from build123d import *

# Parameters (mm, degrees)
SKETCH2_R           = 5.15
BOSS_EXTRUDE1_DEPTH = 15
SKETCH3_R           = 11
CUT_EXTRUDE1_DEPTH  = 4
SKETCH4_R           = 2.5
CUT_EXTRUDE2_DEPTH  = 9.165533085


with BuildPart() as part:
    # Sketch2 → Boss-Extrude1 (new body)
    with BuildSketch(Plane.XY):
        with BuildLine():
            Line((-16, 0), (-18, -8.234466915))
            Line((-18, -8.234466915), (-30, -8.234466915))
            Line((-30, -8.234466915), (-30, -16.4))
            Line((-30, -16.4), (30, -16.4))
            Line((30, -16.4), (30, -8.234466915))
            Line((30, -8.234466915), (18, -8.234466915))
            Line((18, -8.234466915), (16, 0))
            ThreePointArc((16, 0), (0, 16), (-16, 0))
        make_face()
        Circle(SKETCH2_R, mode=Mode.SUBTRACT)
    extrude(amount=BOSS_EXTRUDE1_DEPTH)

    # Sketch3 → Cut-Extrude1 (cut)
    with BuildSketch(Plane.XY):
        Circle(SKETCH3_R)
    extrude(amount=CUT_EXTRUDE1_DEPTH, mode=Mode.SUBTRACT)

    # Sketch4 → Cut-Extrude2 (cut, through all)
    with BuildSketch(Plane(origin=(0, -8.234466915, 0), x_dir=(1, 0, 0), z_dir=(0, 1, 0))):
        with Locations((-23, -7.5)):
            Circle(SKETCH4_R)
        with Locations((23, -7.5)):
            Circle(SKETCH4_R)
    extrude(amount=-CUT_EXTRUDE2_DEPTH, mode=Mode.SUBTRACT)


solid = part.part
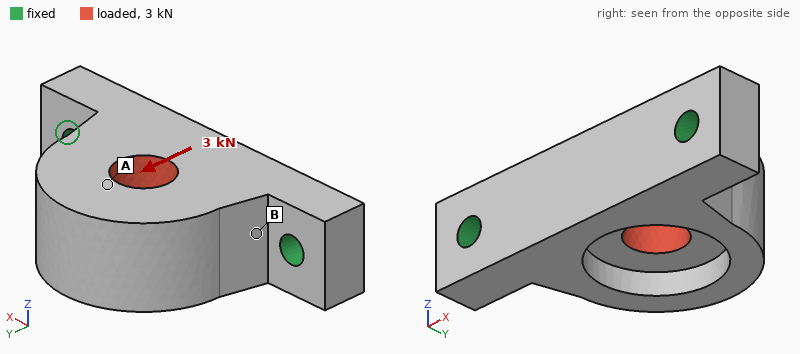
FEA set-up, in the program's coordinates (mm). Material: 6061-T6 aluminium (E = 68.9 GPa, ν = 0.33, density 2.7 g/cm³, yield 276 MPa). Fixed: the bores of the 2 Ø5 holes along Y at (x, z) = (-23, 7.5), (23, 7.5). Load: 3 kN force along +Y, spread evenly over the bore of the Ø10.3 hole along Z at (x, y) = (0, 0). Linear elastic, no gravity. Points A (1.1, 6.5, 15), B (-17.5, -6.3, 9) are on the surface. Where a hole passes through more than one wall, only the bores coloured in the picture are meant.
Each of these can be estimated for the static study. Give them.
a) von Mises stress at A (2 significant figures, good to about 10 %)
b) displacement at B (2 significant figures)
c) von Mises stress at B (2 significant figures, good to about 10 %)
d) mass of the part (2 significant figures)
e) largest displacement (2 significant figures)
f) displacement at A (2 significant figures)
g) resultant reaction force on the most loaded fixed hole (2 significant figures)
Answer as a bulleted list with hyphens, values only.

- 12 MPa
- 6.2 µm
- 33 MPa
- 40 g
- 20 µm
- 16 µm
- 1.6 kN
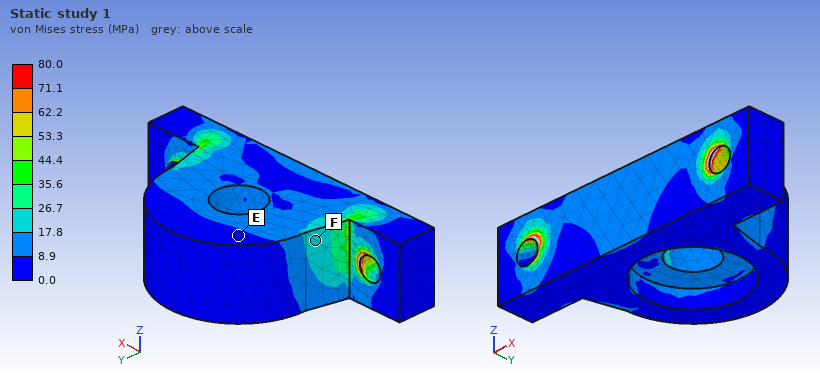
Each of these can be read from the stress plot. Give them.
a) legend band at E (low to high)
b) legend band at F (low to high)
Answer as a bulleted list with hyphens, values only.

- 0.0 to 8.9 MPa
- 17.8 to 26.7 MPa
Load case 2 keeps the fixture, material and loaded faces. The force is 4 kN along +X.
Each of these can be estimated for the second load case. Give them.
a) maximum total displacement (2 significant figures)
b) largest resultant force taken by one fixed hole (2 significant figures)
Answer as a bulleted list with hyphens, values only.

- 13 µm
- 2.3 kN
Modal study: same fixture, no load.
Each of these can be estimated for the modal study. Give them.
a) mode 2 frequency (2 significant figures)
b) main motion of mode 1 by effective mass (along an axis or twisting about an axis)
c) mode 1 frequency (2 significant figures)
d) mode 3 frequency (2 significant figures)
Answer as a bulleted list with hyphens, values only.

- 17 kHz
- along Z
- 6500 Hz
- 18 kHz
